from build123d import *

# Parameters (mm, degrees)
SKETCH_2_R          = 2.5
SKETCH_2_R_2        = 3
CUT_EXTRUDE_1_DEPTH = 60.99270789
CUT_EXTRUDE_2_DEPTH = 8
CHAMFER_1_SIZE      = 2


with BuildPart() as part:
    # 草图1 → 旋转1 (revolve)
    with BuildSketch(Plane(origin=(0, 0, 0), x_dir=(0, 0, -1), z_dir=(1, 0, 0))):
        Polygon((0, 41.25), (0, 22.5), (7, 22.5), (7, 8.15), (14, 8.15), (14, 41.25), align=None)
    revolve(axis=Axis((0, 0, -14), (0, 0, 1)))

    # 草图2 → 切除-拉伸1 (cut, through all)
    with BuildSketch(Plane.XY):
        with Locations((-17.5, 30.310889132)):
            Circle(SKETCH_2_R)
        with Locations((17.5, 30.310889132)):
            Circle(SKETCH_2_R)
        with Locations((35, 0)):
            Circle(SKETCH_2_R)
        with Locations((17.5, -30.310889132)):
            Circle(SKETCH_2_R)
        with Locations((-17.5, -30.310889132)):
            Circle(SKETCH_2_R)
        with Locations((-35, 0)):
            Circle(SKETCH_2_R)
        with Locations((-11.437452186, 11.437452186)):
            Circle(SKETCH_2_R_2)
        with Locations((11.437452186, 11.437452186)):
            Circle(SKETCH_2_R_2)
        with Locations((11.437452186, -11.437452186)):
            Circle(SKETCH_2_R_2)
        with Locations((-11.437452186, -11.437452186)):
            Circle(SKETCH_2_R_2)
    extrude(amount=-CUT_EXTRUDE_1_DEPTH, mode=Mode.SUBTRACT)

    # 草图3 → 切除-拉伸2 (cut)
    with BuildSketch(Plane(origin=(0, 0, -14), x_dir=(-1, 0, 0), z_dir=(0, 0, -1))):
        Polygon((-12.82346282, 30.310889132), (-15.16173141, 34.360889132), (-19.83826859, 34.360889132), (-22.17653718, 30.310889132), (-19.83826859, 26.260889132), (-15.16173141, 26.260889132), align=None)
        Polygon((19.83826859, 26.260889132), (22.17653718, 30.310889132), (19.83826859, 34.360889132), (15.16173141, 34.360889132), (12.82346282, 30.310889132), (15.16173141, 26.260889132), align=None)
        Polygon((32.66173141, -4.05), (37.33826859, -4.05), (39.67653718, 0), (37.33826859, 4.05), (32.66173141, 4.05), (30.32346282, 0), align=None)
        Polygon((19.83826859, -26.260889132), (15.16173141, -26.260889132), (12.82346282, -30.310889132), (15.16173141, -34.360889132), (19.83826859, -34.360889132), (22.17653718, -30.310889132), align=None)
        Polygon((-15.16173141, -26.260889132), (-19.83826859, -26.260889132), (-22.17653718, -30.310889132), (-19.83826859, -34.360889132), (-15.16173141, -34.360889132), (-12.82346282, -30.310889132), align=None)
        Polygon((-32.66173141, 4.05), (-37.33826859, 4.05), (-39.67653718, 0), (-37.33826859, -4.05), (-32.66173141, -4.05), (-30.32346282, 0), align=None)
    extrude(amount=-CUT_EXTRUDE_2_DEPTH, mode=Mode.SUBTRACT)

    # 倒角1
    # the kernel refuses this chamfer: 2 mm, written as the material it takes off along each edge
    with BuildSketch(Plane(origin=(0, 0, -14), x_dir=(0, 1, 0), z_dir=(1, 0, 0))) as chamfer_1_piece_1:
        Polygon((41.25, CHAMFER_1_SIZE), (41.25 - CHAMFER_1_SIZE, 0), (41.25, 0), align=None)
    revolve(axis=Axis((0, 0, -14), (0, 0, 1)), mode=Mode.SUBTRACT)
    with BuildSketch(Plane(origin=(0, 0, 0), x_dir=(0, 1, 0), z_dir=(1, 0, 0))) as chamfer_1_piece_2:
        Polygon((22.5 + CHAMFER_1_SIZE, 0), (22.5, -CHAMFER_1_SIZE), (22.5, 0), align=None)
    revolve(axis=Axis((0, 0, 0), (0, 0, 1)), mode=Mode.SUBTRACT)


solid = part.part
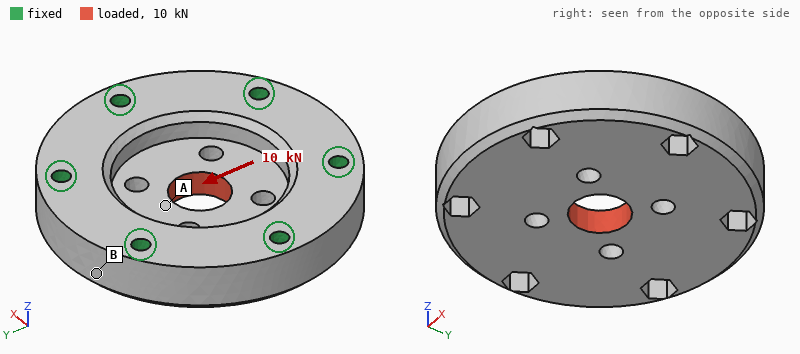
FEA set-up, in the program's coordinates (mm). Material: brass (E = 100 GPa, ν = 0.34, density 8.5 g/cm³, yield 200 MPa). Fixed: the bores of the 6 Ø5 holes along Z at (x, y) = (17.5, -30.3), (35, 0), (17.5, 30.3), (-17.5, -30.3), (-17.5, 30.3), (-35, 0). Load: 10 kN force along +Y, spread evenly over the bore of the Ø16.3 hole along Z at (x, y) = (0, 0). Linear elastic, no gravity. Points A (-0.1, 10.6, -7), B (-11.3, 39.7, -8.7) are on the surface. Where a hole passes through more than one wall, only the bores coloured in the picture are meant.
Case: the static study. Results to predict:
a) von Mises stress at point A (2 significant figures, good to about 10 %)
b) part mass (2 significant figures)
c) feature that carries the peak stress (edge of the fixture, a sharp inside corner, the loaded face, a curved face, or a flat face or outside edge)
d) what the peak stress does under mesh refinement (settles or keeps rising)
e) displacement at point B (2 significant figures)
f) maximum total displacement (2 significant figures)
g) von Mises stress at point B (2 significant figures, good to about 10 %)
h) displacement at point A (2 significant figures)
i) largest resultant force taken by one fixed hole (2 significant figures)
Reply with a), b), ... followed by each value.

a) 26 MPa
b) 490 g
c) edge of the fixture
d) keeps rising
e) 4.2 µm
f) 10 µm
g) 6.7 MPa
h) 8.6 µm
i) 1.9 kN
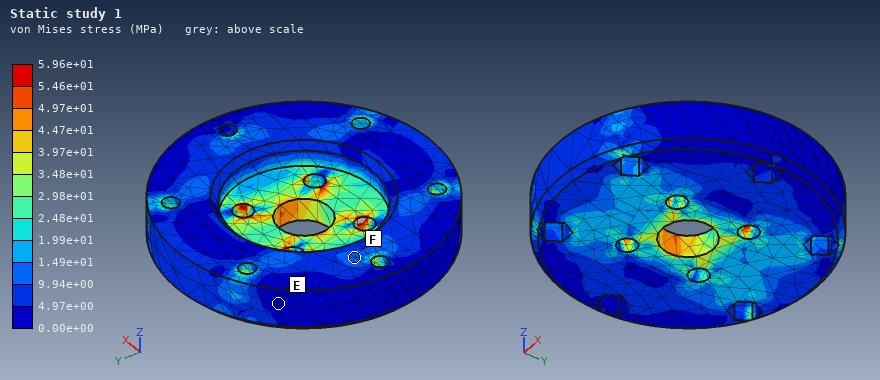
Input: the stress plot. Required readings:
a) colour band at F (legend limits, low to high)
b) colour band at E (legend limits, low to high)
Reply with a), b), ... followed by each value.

a) 9.94e+00 to 1.49e+01 MPa
b) 0.00e+00 to 4.97e+00 MPa
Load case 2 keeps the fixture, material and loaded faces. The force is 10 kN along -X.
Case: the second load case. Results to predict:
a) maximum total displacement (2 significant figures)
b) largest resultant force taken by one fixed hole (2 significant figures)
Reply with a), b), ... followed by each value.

a) 10 µm
b) 2.2 kN
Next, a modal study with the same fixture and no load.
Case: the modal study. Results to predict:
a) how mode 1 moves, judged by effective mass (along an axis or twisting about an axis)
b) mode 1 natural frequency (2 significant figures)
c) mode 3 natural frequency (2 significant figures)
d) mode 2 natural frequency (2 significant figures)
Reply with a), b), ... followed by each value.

a) along Z
b) 11 kHz
c) 14 kHz
d) 14 kHz
